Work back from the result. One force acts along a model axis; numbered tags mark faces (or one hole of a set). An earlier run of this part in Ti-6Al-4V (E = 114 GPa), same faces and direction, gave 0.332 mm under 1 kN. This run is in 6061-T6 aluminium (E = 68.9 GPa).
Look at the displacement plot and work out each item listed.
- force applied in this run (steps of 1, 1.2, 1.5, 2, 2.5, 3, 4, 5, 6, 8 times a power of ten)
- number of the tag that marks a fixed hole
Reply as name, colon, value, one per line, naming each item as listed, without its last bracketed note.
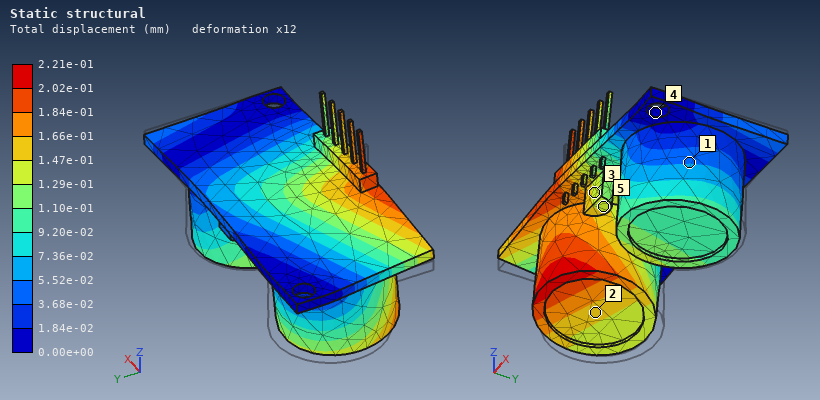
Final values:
force applied in this run: 400 N
number of the tag that marks a fixed hole: 4
